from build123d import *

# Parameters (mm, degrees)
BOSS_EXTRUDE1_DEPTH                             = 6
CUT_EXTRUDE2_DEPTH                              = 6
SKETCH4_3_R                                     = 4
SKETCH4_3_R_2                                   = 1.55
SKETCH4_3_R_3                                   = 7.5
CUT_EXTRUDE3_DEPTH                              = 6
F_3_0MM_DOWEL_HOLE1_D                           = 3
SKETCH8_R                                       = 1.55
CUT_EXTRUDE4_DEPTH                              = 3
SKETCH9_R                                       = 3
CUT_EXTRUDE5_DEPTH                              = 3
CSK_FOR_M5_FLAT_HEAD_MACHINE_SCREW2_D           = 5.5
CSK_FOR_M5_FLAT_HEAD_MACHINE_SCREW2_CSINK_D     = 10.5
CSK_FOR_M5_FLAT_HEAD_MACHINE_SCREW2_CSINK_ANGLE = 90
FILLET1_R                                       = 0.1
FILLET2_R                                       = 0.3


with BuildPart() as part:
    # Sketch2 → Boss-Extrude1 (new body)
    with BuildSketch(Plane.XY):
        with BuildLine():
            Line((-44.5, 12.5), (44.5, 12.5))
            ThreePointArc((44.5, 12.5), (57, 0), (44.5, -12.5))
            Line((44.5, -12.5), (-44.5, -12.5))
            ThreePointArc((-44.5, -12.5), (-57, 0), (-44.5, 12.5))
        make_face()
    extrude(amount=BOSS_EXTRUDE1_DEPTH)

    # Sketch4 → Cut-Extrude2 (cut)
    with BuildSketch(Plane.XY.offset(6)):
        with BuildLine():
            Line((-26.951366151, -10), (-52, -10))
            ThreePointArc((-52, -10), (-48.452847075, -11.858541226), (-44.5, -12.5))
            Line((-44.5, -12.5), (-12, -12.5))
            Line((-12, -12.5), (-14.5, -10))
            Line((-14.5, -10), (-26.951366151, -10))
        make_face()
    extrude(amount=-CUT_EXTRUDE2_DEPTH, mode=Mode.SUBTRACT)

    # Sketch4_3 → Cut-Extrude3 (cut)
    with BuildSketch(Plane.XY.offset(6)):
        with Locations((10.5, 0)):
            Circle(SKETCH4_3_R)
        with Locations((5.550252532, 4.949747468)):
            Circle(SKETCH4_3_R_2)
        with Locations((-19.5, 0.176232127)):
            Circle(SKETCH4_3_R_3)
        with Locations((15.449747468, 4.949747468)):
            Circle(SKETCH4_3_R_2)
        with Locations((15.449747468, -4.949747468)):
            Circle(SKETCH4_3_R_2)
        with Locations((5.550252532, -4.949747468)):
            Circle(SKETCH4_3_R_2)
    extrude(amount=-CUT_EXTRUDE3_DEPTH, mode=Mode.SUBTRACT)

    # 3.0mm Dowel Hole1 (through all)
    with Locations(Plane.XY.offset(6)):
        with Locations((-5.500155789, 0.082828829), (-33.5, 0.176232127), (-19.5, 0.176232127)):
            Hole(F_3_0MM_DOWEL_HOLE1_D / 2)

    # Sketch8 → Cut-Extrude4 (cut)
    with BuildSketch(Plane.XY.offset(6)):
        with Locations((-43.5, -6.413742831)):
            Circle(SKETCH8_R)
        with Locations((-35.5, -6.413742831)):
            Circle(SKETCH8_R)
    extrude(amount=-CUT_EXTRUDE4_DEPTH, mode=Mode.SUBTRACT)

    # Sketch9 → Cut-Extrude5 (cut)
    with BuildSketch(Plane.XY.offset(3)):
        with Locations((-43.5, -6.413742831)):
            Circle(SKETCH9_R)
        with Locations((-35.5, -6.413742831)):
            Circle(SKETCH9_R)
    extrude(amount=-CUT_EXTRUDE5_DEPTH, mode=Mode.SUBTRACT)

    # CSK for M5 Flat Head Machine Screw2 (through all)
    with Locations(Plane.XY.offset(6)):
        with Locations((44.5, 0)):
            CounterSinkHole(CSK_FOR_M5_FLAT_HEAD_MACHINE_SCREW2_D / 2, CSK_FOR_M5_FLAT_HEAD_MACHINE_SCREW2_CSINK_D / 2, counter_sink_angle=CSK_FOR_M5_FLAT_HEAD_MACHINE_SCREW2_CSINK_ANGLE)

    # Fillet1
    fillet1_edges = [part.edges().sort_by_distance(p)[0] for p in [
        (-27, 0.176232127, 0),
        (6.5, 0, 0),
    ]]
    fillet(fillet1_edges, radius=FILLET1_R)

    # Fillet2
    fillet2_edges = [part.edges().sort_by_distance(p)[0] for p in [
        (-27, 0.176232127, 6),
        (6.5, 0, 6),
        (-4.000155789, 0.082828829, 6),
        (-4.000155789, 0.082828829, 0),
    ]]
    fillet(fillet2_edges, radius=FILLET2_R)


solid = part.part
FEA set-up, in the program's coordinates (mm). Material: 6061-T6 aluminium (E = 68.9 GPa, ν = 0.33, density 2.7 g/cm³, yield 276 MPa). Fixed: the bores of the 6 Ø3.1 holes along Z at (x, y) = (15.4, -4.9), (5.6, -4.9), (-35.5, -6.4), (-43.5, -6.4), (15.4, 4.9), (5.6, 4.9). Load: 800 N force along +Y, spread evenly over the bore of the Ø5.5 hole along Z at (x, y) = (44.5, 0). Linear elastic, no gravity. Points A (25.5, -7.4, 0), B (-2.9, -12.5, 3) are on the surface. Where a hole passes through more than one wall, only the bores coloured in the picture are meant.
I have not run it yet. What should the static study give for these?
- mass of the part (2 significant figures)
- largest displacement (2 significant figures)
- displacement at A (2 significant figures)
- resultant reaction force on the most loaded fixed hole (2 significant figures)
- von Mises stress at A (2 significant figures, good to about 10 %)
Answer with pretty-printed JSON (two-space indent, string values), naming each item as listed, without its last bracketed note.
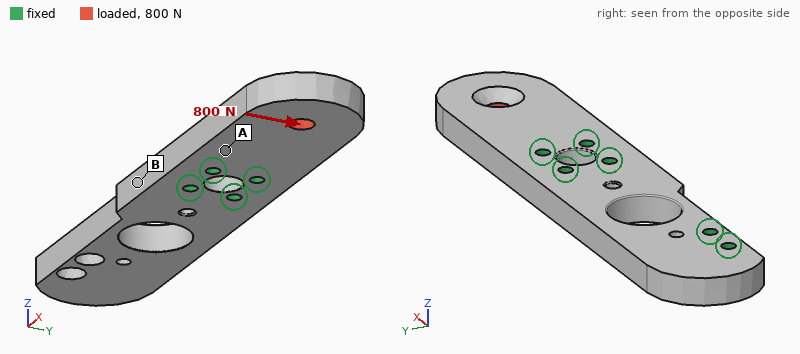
{
  "mass of the part": "37 g",
  "largest displacement": "37 µm",
  "displacement at A": "7.6 µm",
  "resultant reaction force on the most loaded fixed hole": "1.3 kN",
  "von Mises stress at A": "19 MPa"
}
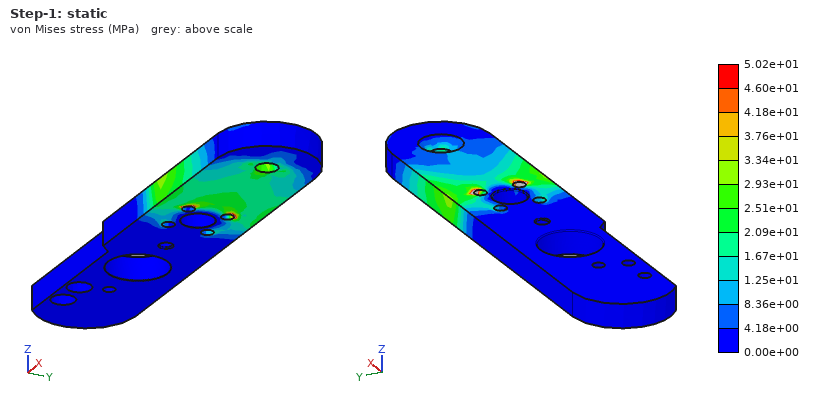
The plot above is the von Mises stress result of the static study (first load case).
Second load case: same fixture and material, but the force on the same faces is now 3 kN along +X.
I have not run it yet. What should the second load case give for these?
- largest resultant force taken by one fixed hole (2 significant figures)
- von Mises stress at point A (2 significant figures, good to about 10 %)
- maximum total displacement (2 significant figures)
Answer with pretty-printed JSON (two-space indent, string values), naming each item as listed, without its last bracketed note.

{
  "largest resultant force taken by one fixed hole": "1.3 kN",
  "von Mises stress at point A": "45 MPa",
  "maximum total displacement": "97 µm"
}
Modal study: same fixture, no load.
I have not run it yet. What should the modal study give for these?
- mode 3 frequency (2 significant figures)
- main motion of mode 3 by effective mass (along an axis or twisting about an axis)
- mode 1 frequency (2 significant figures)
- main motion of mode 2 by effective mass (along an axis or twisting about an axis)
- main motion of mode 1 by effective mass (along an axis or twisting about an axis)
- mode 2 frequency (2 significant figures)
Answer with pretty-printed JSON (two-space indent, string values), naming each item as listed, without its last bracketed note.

{
  "mode 3 frequency": "9500 Hz",
  "main motion of mode 3 by effective mass": "along Y",
  "mode 1 frequency": "3200 Hz",
  "main motion of mode 2 by effective mass": "along Z",
  "main motion of mode 1 by effective mass": "along Z",
  "mode 2 frequency": "7900 Hz"
}
